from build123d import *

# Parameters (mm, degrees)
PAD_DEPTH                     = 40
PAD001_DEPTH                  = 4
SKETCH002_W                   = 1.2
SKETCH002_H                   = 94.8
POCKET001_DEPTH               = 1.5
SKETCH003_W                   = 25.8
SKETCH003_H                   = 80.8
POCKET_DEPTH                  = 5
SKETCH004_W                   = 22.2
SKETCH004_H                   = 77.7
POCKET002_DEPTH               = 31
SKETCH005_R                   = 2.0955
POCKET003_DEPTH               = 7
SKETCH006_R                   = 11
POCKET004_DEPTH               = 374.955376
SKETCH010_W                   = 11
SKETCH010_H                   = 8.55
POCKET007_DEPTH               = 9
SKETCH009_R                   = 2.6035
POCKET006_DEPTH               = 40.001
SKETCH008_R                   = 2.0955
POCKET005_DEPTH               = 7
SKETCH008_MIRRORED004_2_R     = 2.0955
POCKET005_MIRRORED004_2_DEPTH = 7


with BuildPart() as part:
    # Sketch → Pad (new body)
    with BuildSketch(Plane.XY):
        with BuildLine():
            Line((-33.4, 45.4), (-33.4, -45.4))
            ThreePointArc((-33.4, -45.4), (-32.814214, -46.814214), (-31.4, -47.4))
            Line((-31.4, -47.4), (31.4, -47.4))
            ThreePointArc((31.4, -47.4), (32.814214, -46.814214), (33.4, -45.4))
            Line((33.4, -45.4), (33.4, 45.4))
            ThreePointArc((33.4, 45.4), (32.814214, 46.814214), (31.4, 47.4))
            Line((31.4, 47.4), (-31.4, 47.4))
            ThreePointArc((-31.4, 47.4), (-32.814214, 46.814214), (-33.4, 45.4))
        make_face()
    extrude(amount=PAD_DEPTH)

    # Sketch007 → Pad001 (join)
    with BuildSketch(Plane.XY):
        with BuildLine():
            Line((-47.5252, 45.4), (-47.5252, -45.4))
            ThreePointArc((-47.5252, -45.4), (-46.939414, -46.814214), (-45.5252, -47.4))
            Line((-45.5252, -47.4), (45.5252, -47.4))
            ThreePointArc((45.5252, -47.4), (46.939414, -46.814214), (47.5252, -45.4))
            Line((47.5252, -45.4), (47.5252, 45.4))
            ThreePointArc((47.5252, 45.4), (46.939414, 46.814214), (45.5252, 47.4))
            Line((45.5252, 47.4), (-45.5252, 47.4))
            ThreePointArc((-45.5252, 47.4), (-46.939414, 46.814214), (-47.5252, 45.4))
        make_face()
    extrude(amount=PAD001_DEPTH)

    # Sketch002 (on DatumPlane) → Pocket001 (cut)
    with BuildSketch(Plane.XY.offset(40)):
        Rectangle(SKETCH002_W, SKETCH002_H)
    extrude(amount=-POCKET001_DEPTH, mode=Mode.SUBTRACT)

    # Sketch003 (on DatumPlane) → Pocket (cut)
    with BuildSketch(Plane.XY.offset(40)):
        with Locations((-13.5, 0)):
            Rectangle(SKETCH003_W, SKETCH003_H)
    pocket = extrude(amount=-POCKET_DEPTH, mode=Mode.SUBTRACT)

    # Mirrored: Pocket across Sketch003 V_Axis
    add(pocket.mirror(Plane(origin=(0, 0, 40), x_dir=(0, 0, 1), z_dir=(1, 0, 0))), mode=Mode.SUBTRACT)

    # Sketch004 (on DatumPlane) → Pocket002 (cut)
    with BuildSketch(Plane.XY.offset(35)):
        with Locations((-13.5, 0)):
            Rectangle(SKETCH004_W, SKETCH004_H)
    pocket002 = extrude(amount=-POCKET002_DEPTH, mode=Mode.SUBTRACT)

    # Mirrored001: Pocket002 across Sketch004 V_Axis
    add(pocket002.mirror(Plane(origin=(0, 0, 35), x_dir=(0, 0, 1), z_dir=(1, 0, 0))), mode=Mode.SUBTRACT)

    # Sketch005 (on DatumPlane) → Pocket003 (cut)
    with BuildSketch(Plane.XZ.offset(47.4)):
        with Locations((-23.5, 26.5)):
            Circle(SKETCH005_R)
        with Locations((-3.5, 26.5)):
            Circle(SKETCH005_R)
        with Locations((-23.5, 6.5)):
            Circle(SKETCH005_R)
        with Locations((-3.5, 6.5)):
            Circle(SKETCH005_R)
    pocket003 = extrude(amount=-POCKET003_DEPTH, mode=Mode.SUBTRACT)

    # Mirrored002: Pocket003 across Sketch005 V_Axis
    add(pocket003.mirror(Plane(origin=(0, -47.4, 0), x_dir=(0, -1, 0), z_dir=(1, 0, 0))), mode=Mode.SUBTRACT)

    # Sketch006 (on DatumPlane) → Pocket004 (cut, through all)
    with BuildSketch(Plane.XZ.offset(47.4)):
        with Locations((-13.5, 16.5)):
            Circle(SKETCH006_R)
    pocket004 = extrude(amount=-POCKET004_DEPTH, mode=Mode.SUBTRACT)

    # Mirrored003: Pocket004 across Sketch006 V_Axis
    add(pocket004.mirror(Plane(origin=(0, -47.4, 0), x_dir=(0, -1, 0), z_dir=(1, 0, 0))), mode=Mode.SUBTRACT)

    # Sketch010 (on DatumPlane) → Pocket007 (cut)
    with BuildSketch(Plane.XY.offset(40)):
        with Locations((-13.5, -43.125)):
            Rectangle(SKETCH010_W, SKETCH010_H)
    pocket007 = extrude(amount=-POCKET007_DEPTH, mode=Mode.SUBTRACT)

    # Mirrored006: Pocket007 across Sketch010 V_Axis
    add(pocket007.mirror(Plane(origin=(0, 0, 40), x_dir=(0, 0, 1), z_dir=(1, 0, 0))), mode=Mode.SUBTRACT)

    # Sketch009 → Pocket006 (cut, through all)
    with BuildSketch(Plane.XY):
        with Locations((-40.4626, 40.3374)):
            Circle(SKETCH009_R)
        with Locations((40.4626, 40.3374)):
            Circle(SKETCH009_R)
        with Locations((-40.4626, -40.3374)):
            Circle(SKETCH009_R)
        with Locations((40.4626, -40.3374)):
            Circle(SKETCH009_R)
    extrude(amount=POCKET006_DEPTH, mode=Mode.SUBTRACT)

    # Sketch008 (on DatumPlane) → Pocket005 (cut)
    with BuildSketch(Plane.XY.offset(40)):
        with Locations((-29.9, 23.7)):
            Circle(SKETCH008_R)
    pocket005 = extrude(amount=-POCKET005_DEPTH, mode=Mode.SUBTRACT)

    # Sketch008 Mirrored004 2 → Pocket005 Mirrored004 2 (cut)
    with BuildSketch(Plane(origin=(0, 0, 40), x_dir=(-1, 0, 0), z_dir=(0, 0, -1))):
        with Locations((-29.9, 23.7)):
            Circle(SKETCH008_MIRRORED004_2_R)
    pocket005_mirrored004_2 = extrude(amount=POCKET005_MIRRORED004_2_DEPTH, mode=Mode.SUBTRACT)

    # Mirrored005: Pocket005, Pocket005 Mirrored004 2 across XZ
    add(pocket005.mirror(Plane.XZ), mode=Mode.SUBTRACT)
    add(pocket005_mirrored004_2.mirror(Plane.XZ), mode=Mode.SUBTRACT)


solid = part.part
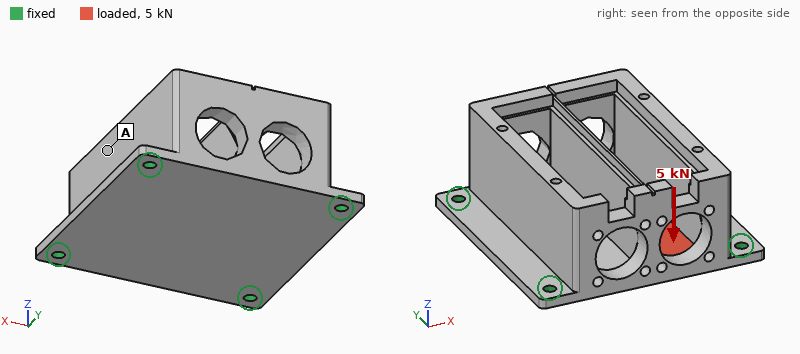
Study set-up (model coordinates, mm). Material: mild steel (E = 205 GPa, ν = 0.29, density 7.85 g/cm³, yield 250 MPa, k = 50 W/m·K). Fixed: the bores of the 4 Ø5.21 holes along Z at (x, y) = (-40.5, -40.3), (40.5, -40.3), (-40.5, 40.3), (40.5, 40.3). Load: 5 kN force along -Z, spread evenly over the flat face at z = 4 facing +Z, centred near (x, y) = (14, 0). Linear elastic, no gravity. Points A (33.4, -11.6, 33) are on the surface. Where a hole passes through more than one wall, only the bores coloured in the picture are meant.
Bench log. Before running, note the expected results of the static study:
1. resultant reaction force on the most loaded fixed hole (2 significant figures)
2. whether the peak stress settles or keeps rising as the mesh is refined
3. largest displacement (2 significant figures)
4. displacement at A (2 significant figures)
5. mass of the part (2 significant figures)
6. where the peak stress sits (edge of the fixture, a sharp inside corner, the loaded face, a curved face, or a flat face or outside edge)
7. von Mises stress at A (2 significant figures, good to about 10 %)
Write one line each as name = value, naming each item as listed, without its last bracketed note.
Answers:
resultant reaction force on the most loaded fixed hole = 1.8 kN
whether the peak stress settles or keeps rising as the mesh is refined = keeps rising
largest displacement = 20 µm
displacement at A = 13 µm
mass of the part = 940 g
where the peak stress sits = edge of the fixture
von Mises stress at A = 14 MPa
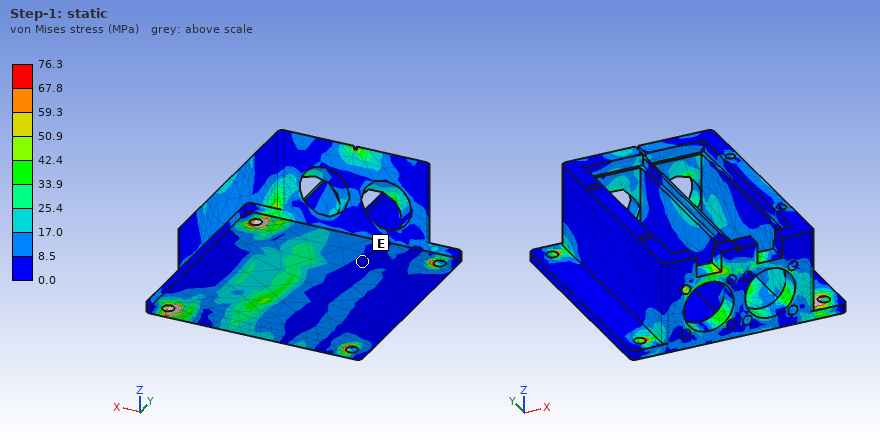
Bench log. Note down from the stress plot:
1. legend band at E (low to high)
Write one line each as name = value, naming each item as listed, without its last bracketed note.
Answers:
legend band at E = 0.0 to 8.5 MPa
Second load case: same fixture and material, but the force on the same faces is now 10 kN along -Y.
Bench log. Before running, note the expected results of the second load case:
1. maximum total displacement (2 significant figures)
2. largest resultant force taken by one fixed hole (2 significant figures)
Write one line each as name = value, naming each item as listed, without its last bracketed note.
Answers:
maximum total displacement = 7.6 µm
largest resultant force taken by one fixed hole = 3.4 kN
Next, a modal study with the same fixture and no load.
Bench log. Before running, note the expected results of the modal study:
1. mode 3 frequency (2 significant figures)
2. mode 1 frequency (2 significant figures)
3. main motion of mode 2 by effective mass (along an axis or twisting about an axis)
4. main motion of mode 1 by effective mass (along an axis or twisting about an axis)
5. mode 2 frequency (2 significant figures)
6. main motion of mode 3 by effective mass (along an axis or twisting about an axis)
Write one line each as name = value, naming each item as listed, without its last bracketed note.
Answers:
mode 3 frequency = 4800 Hz
mode 1 frequency = 4100 Hz
main motion of mode 2 by effective mass = along X
main motion of mode 1 by effective mass = along Z
mode 2 frequency = 4300 Hz
main motion of mode 3 by effective mass = along Y
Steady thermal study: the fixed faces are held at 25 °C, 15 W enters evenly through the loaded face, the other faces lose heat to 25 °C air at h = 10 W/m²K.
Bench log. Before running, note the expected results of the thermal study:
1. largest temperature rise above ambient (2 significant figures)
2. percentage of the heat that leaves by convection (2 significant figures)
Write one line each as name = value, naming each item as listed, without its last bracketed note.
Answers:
largest temperature rise above ambient = 15 K
percentage of the heat that leaves by convection = 24 %
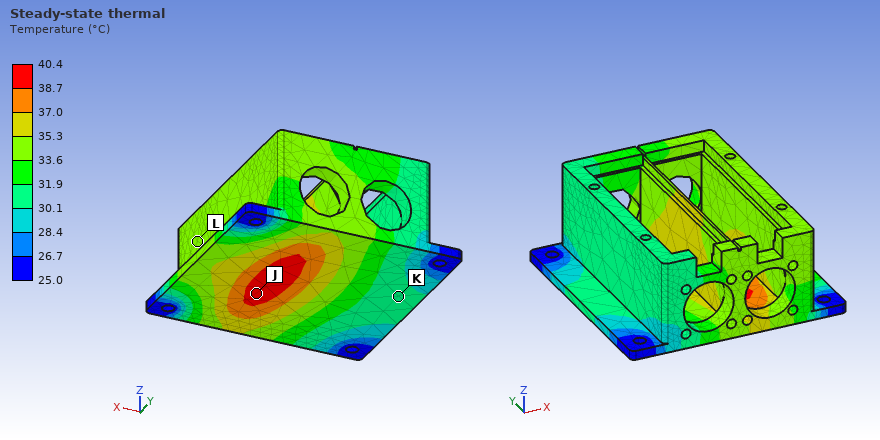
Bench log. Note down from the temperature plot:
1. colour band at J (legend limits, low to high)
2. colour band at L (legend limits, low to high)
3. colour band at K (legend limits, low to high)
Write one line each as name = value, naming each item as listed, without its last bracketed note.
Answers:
colour band at J = 38.7 to 40.4 °C
colour band at L = 33.6 to 35.3 °C
colour band at K = 30.1 to 31.9 °C
